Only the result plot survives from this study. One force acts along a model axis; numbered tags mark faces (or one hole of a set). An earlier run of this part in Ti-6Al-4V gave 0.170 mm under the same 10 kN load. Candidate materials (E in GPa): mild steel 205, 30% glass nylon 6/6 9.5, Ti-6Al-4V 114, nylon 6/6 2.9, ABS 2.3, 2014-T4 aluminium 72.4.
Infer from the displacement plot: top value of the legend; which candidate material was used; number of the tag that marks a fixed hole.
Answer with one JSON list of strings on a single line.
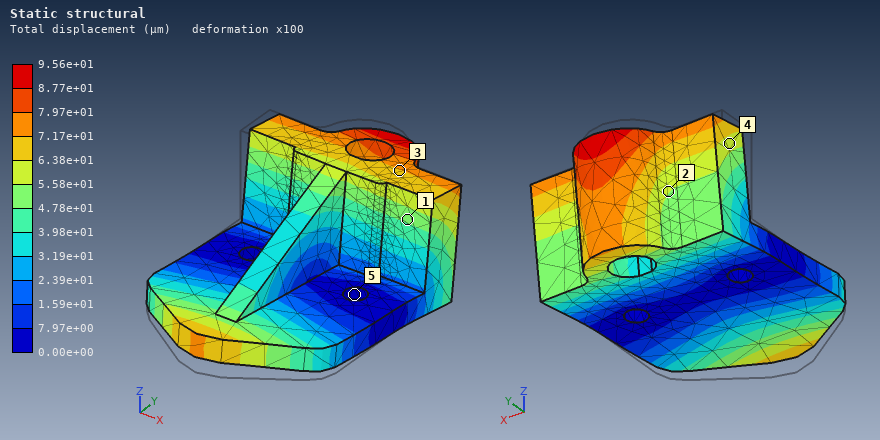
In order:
["9.56e+01 µm", "mild steel", "5"]
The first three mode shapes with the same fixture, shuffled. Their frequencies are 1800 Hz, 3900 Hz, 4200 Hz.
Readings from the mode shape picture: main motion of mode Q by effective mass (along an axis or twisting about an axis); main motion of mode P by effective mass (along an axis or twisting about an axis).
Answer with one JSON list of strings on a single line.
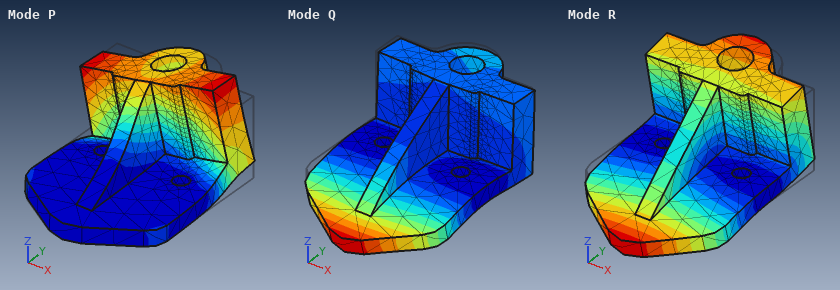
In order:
["along Z", "along X"]
